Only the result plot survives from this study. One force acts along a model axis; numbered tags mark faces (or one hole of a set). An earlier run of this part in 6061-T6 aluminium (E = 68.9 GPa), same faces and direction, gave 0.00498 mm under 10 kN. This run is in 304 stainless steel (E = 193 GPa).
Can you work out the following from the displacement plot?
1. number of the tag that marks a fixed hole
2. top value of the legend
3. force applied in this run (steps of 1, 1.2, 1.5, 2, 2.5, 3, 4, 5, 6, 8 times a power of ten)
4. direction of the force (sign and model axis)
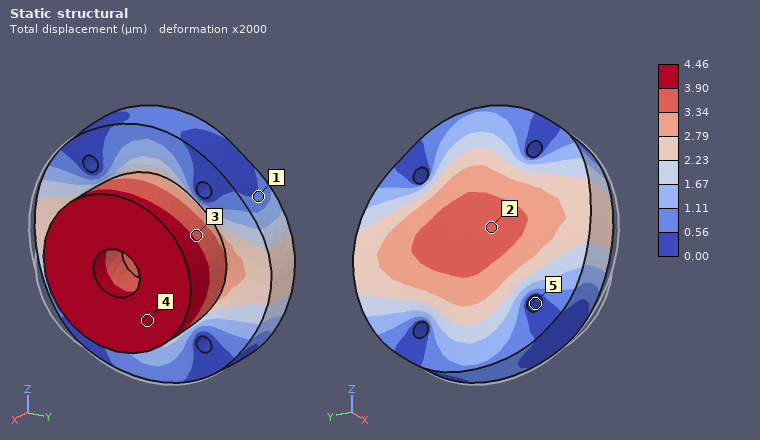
5
4.46 µm
25 kN
-X
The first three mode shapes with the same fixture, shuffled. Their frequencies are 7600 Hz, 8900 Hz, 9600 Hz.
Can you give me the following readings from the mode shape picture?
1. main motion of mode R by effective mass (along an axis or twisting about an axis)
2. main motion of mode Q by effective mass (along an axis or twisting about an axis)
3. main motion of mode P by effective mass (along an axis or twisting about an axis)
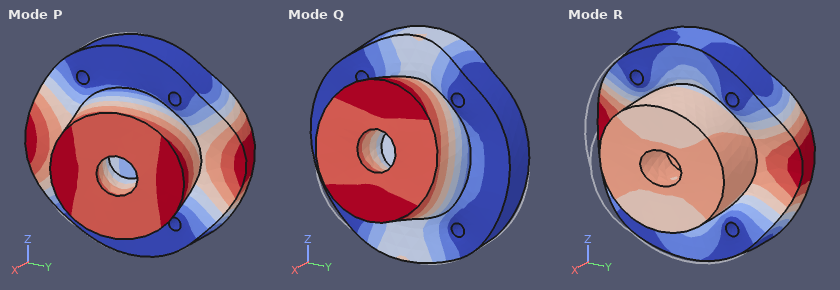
along X
along Z
along Y
